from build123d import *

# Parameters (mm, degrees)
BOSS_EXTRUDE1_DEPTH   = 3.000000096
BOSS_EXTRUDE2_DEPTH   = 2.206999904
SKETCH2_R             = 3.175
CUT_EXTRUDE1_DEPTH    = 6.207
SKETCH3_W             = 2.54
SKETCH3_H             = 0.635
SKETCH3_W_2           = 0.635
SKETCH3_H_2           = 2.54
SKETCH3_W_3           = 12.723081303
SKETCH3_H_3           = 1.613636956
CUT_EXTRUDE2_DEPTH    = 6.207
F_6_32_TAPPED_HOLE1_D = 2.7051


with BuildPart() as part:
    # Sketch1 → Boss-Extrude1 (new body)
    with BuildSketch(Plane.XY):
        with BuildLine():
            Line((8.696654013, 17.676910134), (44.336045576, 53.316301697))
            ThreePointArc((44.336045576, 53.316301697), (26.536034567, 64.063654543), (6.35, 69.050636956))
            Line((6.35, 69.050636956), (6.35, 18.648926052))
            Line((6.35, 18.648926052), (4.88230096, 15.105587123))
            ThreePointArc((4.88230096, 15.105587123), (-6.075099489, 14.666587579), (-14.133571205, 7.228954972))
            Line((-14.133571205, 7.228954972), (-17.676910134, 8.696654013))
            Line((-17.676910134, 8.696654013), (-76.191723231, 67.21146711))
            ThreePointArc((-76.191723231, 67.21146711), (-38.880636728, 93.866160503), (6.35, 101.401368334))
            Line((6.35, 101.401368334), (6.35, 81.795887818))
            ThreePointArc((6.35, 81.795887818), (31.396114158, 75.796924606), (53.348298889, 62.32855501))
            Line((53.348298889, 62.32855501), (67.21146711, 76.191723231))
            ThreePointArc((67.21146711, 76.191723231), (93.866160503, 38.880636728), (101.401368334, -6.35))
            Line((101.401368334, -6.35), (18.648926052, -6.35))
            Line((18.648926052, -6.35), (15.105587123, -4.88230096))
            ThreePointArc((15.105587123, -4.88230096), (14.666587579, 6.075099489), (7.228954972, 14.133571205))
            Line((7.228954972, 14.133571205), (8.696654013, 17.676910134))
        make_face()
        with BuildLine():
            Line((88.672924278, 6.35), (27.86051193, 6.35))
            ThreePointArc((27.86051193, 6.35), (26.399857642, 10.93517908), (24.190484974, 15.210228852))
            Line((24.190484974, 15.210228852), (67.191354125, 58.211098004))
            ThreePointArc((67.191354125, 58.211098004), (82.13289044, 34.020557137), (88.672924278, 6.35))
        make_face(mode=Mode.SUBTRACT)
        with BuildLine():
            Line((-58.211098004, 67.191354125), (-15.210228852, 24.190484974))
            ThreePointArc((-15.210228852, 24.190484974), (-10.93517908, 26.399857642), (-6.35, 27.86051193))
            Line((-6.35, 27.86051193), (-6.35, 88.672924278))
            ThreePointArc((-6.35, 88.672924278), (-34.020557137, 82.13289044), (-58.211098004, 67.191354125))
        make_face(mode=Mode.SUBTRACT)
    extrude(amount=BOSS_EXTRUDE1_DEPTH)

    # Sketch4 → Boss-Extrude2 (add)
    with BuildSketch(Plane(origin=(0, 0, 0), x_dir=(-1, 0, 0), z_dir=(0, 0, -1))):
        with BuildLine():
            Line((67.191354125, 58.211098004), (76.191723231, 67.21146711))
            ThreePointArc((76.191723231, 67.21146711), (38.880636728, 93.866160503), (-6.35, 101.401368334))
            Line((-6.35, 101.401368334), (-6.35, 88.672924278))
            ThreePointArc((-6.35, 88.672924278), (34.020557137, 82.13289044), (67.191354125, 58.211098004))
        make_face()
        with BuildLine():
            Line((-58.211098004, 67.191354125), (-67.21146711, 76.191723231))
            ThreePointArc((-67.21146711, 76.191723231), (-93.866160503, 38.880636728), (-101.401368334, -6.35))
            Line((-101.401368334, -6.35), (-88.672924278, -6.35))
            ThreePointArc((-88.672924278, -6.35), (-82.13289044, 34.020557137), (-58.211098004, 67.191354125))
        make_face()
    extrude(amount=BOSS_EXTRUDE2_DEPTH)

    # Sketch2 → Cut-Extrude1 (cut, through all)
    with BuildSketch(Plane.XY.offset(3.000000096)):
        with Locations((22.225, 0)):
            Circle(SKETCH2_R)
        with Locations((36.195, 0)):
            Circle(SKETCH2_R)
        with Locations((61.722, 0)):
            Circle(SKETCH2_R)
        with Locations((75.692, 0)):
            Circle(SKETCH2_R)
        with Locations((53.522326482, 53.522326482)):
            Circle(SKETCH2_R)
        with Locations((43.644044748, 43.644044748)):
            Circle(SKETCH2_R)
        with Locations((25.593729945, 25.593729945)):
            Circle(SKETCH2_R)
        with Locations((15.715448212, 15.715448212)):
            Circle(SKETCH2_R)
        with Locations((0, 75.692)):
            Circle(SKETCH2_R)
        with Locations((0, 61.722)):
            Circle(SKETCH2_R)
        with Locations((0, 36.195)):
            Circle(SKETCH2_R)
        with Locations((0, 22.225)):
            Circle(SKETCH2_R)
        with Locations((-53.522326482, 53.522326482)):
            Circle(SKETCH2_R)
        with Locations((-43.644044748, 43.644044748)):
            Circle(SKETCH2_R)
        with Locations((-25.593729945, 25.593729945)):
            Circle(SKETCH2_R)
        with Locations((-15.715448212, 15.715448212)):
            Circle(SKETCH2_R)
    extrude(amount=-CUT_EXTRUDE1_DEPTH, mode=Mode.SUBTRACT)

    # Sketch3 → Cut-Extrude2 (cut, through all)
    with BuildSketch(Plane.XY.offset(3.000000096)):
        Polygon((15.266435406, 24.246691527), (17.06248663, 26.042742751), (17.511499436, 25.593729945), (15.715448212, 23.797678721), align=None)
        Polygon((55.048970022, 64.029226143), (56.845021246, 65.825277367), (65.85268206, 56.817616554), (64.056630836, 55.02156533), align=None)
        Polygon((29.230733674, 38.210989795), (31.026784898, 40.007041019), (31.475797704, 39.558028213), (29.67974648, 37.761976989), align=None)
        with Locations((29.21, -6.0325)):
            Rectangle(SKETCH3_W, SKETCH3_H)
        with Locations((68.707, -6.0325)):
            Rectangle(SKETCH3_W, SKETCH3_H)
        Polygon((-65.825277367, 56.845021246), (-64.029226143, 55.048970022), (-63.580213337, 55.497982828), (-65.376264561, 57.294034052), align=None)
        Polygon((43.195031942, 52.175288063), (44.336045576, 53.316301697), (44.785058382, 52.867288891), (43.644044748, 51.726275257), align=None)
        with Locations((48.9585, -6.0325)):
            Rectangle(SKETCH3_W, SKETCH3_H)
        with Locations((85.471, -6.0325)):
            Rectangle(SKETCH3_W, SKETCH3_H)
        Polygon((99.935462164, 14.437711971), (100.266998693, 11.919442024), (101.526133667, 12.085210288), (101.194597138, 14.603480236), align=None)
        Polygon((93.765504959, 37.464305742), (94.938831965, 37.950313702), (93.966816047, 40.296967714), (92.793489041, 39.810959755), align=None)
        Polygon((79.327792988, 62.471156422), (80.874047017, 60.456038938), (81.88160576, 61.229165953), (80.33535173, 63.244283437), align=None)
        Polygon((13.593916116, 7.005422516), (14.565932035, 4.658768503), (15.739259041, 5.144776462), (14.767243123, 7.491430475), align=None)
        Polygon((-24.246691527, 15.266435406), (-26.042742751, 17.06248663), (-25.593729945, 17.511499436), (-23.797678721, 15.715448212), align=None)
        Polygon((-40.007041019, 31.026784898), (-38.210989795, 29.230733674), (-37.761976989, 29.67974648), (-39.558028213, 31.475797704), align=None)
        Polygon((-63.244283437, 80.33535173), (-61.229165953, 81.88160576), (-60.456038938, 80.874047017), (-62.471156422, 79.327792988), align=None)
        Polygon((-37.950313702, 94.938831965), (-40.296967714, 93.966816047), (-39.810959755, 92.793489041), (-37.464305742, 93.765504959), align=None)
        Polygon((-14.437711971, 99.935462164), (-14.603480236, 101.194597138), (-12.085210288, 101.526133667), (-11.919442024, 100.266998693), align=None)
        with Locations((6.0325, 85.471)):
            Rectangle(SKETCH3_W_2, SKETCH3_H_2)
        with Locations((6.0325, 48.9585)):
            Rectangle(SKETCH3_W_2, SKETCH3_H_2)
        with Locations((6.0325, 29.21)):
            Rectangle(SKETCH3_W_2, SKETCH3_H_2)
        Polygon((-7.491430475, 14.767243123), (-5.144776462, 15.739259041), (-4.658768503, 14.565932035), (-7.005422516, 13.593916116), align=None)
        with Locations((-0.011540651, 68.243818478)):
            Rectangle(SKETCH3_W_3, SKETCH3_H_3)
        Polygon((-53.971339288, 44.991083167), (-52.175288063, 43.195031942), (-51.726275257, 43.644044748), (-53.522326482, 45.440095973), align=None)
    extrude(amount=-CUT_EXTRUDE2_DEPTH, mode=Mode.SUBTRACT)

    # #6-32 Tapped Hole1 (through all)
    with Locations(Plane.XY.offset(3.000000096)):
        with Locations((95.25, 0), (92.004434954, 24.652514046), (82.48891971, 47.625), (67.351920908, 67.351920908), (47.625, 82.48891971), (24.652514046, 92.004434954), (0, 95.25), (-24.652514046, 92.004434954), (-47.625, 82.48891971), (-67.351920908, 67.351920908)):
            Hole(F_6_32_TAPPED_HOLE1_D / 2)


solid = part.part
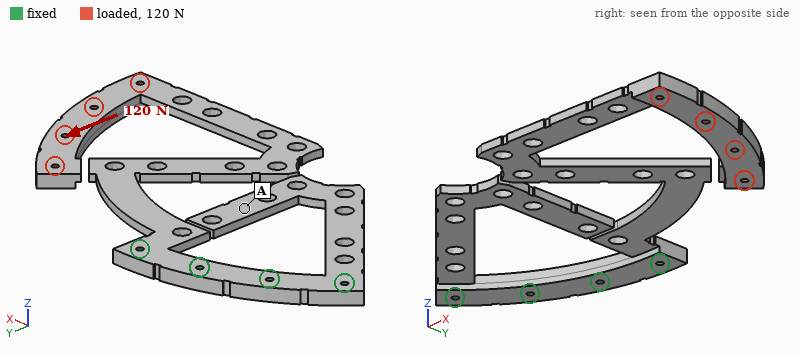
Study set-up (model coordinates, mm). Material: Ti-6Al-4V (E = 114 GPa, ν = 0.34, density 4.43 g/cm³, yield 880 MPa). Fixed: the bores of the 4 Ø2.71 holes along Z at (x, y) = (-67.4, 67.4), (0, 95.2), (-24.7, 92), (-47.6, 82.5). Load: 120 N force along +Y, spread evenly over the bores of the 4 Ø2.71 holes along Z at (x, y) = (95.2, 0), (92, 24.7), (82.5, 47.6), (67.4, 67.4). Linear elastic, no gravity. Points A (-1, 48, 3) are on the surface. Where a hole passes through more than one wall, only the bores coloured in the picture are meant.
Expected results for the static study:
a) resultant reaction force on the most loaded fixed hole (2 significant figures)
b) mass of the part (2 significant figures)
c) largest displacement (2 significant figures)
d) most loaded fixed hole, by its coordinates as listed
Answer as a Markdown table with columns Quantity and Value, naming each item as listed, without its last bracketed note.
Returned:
| Quantity | Value |
|---|---|
| resultant reaction force on the most loaded fixed hole | 480 N |
| mass of the part | 100 g |
| largest displacement | 2.4 mm |
| most loaded fixed hole, by its coordinates as listed | (0, 95.2) |
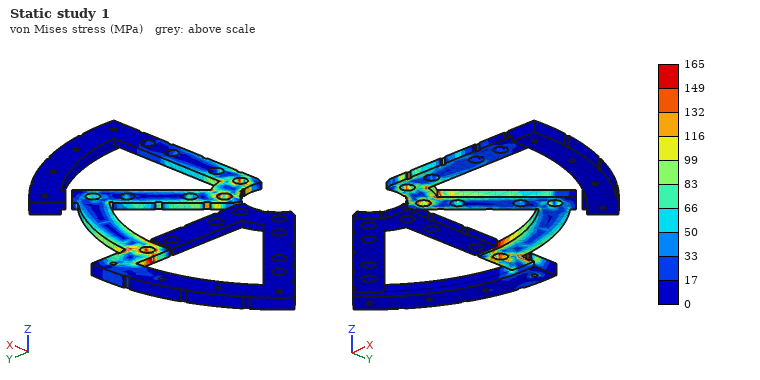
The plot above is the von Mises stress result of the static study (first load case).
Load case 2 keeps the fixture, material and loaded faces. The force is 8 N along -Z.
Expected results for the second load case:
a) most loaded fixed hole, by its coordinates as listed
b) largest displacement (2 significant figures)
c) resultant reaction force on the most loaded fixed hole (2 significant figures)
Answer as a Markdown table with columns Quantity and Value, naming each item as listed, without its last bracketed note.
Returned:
| Quantity | Value |
|---|---|
| most loaded fixed hole, by its coordinates as listed | (0, 95.2) |
| largest displacement | 2.2 mm |
| resultant reaction force on the most loaded fixed hole | 23 N |
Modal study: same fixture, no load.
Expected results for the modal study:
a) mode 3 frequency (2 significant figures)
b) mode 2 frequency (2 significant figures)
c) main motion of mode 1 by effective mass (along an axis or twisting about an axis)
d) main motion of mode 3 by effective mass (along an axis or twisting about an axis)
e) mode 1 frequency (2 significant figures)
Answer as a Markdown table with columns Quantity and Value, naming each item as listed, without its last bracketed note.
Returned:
| Quantity | Value |
|---|---|
| mode 3 frequency | 210 Hz |
| mode 2 frequency | 120 Hz |
| main motion of mode 1 by effective mass | along Z |
| main motion of mode 3 by effective mass | along Y |
| mode 1 frequency | 59 Hz |
